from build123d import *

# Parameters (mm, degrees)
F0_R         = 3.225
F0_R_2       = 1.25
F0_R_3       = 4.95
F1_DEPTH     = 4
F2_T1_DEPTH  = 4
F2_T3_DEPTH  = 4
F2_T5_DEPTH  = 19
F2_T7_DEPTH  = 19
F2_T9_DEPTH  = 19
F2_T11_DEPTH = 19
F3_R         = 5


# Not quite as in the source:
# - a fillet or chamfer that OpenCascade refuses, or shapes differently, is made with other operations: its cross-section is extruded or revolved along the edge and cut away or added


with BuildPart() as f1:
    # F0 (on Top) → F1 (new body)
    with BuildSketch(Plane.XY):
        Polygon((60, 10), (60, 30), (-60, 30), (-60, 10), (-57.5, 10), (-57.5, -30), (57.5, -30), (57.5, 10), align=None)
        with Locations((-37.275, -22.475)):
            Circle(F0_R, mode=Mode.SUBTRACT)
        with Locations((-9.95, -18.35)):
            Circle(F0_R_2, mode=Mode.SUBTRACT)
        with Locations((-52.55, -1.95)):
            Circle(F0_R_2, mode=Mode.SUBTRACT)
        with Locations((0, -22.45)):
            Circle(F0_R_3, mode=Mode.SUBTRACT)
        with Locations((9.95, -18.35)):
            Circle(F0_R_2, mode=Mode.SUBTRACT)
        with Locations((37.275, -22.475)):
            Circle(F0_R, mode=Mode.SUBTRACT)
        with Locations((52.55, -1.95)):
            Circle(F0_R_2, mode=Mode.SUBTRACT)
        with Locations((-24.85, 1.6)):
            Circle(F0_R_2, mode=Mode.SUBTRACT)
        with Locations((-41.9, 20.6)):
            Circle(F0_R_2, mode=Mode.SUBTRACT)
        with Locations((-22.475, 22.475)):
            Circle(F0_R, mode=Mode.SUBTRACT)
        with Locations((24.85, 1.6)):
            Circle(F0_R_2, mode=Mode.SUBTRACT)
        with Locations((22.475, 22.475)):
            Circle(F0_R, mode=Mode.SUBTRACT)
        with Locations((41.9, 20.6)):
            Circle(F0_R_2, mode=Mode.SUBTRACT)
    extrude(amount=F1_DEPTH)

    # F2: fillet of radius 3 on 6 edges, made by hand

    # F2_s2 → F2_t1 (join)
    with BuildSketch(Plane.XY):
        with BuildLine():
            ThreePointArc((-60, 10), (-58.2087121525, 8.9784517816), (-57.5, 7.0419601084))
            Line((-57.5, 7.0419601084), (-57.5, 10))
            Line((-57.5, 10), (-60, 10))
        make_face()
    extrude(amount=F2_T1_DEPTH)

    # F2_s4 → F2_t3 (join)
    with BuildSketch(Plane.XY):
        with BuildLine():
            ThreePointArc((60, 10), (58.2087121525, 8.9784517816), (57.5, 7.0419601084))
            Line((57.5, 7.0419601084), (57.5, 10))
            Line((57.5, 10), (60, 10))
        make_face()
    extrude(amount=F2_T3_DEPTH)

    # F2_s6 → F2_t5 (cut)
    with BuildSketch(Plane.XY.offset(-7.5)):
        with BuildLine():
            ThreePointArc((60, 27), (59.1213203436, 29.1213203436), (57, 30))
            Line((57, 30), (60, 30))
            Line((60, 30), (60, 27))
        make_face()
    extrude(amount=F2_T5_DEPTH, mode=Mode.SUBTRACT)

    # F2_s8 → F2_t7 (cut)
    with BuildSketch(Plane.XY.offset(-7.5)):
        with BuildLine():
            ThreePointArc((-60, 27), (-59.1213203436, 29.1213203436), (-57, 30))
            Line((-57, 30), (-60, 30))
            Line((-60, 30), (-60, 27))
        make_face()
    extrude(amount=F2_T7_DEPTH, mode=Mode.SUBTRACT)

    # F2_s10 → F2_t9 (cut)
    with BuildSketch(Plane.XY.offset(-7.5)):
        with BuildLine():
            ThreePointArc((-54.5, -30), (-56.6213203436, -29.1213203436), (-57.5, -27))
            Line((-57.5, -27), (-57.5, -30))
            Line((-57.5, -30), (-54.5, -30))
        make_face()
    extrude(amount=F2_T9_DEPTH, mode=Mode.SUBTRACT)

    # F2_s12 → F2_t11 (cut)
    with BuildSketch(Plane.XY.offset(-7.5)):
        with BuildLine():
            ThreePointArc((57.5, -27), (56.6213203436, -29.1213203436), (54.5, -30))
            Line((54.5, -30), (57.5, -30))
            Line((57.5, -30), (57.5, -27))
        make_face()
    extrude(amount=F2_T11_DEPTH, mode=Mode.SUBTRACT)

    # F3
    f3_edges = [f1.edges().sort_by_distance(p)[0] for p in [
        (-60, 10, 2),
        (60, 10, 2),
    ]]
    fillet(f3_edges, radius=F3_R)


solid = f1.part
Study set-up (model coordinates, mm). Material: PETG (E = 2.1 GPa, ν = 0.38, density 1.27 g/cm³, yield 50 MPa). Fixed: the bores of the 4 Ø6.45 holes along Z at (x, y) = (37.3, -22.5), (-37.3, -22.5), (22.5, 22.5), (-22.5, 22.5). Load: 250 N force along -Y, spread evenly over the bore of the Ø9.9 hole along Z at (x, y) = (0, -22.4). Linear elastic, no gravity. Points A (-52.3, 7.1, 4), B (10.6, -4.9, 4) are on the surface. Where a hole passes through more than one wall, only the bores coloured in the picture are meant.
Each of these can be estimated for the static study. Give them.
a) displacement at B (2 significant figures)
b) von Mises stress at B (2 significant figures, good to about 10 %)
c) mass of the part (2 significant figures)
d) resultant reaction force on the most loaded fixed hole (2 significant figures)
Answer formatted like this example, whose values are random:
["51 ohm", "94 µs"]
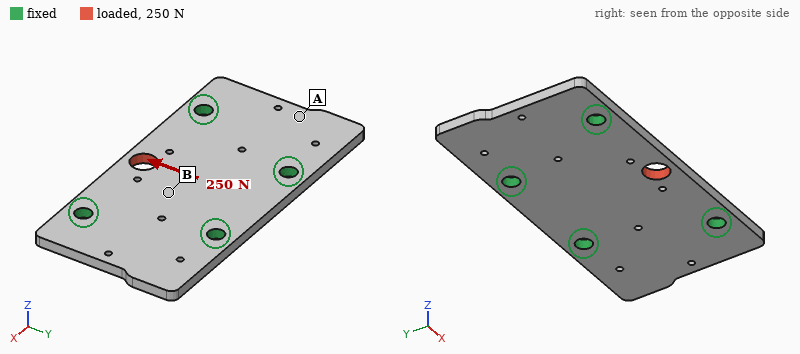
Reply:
["18 µm", "1.5 MPa", "34 g", "96 N"]
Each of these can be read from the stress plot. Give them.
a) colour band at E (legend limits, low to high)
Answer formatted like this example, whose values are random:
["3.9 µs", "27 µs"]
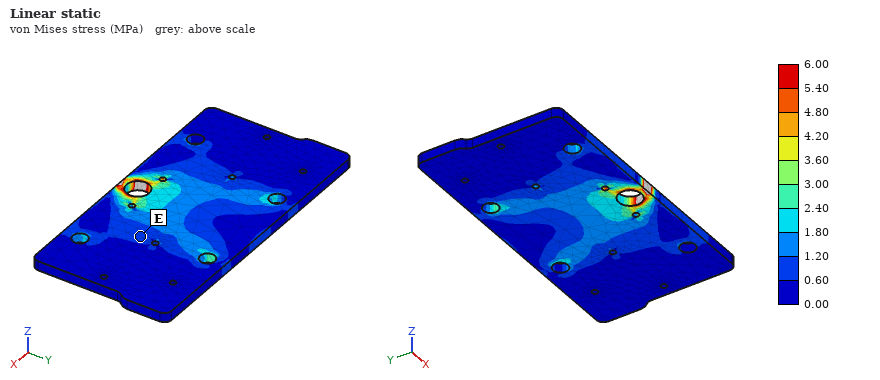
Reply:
["0.60 to 1.20 MPa"]
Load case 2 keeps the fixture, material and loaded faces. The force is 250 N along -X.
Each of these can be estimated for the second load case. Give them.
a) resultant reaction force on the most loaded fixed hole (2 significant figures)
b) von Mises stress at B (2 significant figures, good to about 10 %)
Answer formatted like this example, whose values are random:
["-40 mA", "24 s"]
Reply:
["100 N", "0.45 MPa"]
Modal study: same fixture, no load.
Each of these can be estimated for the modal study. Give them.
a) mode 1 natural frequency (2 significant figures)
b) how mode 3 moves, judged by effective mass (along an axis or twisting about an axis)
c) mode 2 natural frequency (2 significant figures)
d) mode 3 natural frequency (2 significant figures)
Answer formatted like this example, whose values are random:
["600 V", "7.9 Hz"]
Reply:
["830 Hz", "along Z", "850 Hz", "1200 Hz"]
